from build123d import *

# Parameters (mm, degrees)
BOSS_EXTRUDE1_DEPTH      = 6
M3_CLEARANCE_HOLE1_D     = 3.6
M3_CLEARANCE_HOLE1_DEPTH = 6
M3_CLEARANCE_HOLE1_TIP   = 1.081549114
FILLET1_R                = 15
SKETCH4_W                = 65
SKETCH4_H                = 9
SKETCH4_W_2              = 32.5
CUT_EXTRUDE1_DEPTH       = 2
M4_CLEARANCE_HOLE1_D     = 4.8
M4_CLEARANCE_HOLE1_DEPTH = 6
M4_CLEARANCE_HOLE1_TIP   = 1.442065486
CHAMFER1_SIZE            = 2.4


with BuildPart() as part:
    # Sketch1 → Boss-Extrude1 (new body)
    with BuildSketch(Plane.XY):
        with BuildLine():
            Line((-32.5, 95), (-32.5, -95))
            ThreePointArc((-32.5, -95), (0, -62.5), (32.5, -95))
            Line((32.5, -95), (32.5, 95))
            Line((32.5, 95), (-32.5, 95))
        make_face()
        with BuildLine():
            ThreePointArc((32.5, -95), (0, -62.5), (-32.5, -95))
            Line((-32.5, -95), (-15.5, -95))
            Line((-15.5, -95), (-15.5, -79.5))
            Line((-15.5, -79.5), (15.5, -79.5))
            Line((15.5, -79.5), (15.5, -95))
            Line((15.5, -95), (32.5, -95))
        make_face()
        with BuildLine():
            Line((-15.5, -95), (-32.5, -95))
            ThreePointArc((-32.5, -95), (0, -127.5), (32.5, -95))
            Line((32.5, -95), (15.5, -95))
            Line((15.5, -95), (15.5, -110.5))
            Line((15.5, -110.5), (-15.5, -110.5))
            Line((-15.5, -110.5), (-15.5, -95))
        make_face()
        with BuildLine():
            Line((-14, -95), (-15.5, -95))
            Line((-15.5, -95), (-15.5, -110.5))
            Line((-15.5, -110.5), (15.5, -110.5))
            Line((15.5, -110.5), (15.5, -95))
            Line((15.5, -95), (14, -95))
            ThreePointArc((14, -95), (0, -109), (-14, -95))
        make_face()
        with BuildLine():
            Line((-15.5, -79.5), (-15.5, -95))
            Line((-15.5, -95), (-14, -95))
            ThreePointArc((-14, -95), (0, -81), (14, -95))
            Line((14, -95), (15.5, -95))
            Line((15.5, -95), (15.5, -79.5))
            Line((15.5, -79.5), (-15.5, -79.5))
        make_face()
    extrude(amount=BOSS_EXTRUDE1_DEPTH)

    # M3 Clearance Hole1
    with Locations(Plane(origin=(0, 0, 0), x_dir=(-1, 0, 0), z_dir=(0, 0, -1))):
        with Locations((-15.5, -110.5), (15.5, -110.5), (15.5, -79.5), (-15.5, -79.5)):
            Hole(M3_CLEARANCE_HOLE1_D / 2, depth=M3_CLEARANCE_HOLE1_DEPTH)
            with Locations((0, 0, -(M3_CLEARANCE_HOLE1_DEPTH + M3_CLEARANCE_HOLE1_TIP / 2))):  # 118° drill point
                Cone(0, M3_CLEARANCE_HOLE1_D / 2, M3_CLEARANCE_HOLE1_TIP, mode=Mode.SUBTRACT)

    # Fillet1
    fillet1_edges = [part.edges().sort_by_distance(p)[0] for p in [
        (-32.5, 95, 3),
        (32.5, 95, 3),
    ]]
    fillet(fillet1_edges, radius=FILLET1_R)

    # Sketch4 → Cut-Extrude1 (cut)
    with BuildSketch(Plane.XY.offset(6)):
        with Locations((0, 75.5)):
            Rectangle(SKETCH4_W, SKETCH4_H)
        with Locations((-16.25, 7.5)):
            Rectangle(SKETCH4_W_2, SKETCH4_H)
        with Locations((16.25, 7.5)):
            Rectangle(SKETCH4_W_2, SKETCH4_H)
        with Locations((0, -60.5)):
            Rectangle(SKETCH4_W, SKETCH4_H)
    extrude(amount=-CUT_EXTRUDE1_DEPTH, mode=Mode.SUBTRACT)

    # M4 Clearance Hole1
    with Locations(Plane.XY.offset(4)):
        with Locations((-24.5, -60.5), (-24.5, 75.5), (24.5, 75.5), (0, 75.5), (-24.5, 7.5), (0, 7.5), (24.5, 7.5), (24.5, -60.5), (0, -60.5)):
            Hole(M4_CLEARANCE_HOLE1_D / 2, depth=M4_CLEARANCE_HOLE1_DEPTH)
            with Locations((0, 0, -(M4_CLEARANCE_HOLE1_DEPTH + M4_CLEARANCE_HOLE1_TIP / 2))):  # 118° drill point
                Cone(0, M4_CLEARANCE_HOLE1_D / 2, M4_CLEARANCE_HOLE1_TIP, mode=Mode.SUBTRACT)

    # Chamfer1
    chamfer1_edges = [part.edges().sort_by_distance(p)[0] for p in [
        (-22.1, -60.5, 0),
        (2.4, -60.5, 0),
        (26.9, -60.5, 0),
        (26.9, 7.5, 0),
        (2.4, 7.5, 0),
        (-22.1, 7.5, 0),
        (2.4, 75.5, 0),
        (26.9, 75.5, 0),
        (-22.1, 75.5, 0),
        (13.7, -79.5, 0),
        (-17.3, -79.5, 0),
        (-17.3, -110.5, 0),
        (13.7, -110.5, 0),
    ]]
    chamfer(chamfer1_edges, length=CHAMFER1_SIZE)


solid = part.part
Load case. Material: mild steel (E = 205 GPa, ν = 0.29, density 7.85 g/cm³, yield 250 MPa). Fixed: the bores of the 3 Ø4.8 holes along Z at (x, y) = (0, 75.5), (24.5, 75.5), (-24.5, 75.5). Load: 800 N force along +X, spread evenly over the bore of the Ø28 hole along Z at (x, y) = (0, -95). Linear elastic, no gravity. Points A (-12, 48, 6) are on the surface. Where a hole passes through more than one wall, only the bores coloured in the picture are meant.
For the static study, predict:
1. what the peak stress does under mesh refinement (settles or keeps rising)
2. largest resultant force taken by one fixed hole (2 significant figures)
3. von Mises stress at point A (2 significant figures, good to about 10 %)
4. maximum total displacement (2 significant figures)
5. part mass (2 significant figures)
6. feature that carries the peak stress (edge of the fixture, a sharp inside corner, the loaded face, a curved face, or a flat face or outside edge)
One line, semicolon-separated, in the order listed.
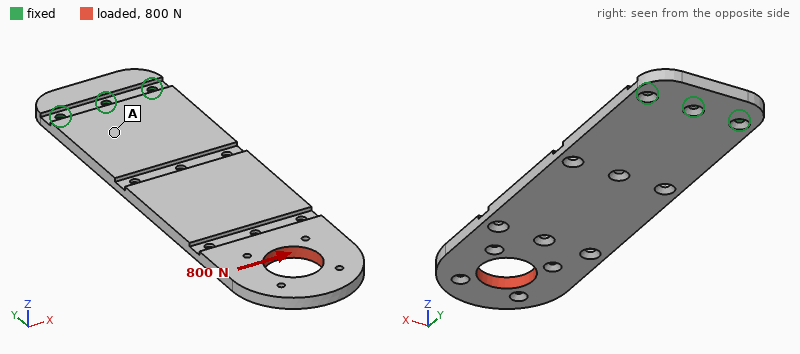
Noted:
keeps rising; 2.7 kN; 9.3 MPa; 88 µm; 590 g; edge of the fixture
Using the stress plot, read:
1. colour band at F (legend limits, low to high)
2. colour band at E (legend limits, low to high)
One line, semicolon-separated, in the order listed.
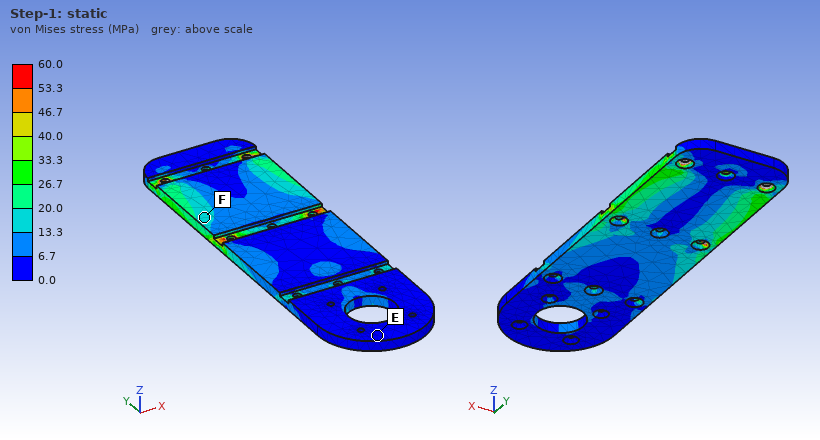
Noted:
13.3 to 20.0 MPa; 0.0 to 6.7 MPa
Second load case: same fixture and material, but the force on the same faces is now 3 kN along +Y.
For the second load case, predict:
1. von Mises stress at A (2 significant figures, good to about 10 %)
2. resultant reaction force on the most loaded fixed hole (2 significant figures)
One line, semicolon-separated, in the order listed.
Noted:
7.6 MPa; 1.0 kN
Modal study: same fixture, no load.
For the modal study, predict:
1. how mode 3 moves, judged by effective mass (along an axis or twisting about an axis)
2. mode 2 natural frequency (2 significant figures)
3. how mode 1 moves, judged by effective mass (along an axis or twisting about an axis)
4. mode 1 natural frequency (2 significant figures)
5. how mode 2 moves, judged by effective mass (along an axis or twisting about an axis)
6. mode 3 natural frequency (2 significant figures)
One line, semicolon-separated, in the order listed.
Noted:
twisting about Y; 600 Hz; along Z; 100 Hz; along Z; 750 Hz
